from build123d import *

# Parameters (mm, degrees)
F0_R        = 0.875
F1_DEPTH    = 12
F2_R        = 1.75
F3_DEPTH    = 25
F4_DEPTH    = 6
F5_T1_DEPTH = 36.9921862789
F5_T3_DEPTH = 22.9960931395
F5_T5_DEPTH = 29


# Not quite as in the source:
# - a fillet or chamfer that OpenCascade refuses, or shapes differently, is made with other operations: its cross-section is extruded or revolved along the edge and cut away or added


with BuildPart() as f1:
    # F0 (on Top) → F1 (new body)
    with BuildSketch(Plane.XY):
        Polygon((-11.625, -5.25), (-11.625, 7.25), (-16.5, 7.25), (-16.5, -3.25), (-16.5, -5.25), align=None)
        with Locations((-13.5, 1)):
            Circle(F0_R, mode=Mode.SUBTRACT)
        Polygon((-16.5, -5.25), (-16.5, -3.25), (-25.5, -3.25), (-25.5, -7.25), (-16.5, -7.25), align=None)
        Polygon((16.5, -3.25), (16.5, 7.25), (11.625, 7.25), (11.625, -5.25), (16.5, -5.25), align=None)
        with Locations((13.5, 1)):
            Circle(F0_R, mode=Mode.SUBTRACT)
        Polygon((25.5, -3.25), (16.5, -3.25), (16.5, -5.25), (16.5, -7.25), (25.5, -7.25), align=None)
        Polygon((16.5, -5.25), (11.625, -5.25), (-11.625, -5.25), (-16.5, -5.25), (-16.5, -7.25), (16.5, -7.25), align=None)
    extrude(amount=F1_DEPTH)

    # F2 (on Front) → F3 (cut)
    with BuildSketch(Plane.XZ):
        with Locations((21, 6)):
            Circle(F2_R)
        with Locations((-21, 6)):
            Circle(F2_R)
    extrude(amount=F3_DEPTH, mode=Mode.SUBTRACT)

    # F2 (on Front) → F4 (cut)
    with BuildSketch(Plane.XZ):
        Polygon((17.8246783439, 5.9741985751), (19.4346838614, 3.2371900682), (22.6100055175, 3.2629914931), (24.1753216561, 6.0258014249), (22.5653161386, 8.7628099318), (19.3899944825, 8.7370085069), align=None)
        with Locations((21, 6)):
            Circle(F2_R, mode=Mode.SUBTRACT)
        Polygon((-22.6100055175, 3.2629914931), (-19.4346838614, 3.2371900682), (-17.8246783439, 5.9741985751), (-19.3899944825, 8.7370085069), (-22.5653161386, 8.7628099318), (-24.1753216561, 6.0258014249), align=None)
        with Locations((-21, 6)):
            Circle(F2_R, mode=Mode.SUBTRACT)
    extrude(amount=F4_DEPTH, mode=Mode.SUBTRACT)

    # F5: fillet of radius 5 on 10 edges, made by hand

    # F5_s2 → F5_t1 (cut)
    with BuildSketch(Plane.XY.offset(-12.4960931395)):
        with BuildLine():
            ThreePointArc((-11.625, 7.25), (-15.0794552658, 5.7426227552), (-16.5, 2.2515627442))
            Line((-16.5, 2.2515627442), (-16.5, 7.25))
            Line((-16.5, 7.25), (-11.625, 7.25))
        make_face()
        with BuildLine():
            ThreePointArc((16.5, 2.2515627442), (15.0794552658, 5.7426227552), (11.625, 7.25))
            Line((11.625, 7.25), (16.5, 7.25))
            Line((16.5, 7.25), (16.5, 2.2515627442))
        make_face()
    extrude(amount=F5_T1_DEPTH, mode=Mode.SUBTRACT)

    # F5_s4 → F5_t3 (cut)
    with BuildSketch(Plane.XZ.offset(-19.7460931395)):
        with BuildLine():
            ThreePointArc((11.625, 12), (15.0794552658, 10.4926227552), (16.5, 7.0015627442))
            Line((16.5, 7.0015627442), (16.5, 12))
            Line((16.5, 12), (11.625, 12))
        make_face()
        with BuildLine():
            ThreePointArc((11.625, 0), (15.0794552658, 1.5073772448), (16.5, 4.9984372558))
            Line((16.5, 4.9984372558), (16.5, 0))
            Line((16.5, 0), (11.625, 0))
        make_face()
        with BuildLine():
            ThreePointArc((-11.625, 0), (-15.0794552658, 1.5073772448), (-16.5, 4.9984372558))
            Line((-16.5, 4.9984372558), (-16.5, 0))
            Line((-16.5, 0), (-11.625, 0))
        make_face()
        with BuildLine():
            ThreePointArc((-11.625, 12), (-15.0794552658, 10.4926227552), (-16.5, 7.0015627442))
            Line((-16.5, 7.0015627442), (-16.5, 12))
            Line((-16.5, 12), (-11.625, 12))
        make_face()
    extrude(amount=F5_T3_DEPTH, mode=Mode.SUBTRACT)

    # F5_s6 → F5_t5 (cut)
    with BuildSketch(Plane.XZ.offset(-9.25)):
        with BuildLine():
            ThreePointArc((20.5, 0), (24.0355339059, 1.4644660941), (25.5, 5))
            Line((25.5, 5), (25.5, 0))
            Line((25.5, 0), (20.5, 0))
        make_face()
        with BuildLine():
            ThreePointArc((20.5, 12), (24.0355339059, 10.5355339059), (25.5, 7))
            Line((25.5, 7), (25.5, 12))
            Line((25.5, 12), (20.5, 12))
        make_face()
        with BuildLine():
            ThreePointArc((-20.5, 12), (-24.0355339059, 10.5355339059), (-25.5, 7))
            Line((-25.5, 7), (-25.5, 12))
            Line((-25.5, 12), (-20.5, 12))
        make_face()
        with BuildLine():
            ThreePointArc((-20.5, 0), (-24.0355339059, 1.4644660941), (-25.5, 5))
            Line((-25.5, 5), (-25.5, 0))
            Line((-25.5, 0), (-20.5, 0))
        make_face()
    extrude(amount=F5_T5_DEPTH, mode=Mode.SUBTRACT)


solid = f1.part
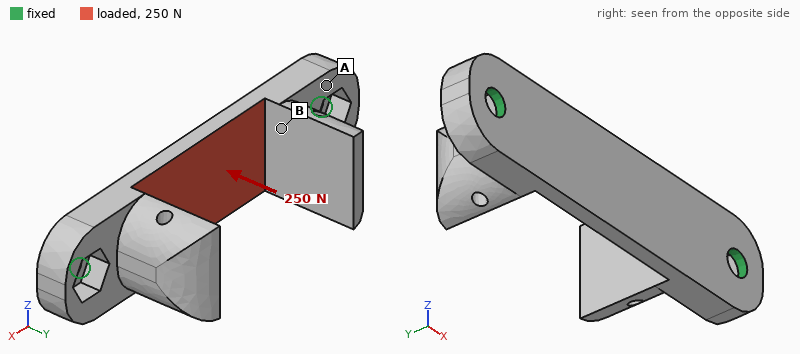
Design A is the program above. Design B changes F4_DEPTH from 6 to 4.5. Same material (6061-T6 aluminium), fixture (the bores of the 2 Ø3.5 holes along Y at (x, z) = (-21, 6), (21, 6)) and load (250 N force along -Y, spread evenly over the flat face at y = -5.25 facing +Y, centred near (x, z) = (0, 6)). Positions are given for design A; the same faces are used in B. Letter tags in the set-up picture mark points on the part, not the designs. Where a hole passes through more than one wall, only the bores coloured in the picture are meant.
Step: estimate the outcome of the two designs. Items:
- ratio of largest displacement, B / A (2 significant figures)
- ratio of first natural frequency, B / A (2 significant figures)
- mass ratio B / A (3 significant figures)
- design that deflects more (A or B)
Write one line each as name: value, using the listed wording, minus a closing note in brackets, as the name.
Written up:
ratio of largest displacement, B / A: 0.58
ratio of first natural frequency, B / A: 1.5
mass ratio B / A: 1.02
design that deflects more: A
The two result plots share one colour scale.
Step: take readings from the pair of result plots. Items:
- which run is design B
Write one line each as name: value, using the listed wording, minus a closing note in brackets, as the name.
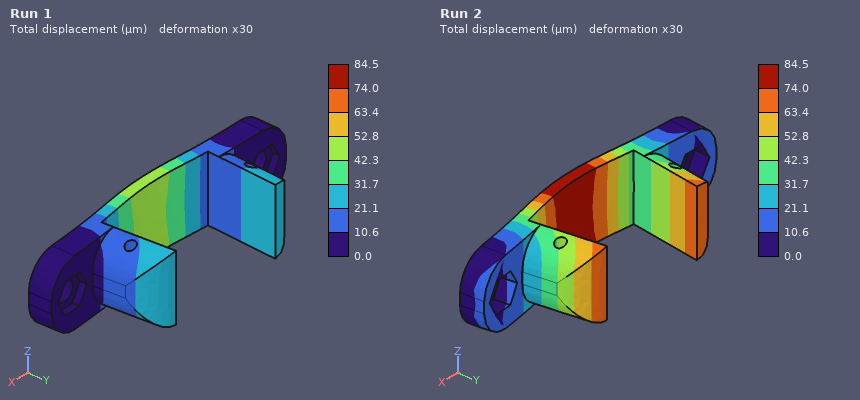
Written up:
which run is design B: Run 1
